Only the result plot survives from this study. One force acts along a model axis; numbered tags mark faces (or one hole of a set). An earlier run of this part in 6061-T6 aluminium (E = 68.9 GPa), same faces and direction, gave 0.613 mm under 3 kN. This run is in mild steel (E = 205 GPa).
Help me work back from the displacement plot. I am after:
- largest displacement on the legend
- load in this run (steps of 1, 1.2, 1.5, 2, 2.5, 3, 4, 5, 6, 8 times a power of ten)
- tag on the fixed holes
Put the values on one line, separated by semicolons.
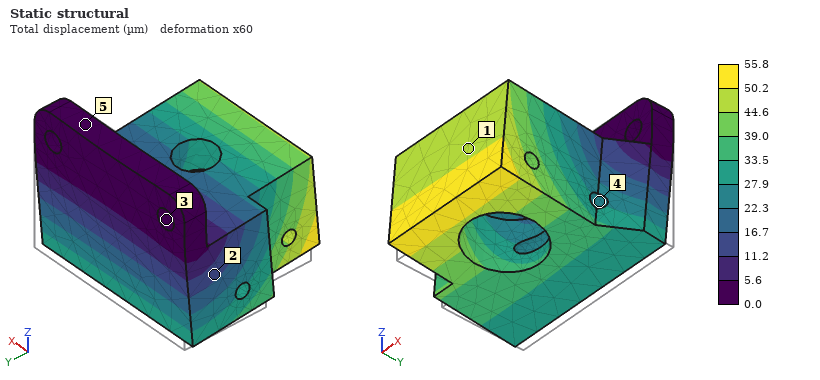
55.8 µm; 800 N; 3
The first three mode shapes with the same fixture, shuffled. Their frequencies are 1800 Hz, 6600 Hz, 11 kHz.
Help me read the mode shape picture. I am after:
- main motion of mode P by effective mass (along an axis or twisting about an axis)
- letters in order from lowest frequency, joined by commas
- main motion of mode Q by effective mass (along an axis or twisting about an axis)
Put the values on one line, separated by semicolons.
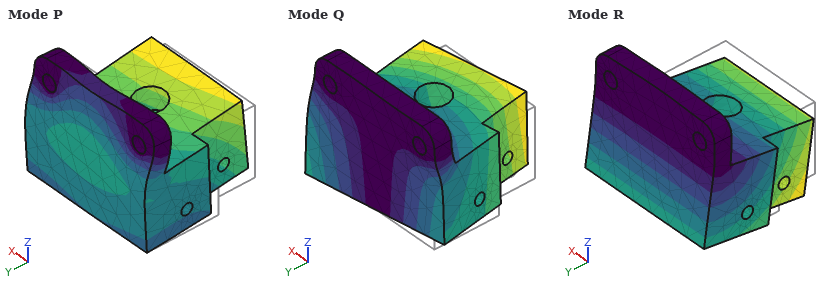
along Y; R, Q, P; along X
